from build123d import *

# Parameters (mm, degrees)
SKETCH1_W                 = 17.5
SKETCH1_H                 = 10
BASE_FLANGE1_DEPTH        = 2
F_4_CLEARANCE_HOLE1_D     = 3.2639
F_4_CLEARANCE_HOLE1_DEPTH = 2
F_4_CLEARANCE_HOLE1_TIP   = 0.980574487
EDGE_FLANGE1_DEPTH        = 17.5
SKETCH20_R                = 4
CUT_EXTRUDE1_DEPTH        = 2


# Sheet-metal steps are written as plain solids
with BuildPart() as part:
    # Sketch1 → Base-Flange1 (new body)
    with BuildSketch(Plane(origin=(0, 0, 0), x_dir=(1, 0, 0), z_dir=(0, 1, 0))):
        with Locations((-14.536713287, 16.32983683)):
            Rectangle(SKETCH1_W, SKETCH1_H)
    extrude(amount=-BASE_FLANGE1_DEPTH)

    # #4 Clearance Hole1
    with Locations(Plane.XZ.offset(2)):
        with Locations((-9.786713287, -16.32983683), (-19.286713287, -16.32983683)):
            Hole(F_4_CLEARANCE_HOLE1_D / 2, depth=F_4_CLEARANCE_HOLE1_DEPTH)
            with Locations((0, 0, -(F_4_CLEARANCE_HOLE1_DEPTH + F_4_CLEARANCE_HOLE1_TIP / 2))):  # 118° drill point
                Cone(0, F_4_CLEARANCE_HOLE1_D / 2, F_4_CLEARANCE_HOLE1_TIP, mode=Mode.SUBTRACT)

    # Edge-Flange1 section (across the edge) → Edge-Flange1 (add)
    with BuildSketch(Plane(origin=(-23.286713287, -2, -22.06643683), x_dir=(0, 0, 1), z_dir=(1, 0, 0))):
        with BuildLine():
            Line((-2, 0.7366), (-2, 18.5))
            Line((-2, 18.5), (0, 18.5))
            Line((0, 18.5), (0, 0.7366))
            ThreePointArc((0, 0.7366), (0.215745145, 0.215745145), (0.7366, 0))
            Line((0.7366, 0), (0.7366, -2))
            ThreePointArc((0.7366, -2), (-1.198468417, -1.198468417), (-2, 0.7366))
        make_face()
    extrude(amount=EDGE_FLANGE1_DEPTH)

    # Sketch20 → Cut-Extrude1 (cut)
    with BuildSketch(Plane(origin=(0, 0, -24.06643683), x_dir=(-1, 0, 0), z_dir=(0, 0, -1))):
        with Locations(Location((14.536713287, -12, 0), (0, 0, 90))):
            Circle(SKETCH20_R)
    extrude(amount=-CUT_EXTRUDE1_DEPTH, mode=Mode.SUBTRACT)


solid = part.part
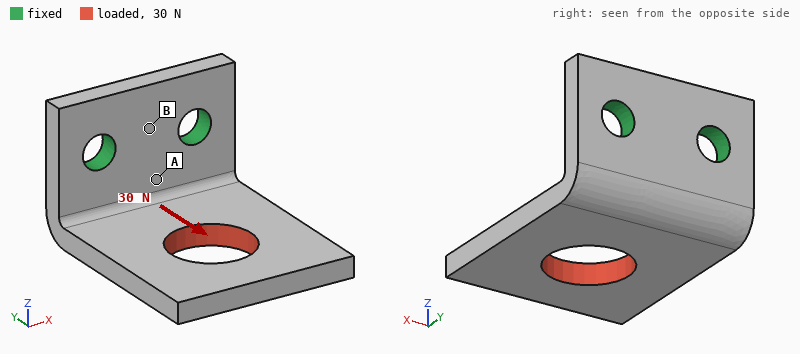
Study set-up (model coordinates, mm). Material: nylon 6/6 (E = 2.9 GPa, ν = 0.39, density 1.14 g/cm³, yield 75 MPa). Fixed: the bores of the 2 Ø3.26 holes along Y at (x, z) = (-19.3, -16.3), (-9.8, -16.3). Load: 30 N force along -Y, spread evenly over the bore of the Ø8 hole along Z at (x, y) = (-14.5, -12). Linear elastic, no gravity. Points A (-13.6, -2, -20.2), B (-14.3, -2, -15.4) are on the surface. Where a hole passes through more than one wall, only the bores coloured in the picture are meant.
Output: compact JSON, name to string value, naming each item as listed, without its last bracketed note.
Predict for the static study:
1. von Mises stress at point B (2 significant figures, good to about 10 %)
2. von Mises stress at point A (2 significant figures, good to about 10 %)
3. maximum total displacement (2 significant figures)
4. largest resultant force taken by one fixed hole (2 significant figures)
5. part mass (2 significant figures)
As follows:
{"von Mises stress at point B": "2.4 MPa", "von Mises stress at point A": "5.8 MPa", "maximum total displacement": "0.29 mm", "largest resultant force taken by one fixed hole": "15 N", "part mass": "1.1 g"}
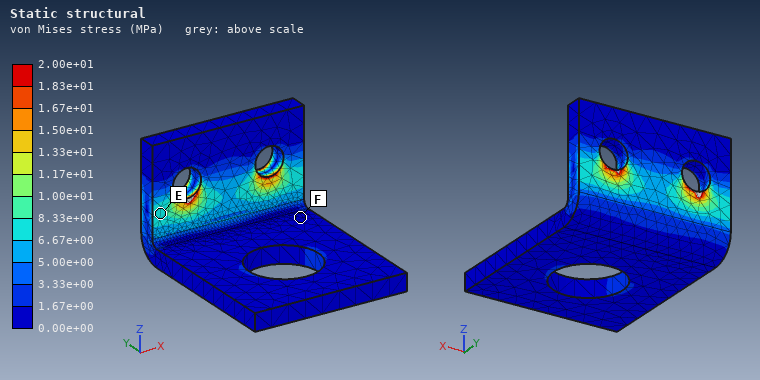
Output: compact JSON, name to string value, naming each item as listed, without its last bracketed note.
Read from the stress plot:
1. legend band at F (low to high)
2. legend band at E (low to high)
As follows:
{"legend band at F": "0.00e+00 to 1.67e+00 MPa", "legend band at E": "6.67e+00 to 8.33e+00 MPa"}
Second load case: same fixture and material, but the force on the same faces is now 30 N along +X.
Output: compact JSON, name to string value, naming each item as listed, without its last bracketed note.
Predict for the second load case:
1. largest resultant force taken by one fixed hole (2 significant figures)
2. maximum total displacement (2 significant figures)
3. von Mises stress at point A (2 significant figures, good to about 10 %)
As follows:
{"largest resultant force taken by one fixed hole": "36 N", "maximum total displacement": "0.30 mm", "von Mises stress at point A": "9.5 MPa"}
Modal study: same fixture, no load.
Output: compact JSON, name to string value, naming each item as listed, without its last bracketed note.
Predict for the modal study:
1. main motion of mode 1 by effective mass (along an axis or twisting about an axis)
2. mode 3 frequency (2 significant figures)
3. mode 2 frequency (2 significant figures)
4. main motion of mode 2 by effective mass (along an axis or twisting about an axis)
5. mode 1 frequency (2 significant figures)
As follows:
{"main motion of mode 1 by effective mass": "along Z", "mode 3 frequency": "3200 Hz", "mode 2 frequency": "2300 Hz", "main motion of mode 2 by effective mass": "along X", "mode 1 frequency": "1000 Hz"}
